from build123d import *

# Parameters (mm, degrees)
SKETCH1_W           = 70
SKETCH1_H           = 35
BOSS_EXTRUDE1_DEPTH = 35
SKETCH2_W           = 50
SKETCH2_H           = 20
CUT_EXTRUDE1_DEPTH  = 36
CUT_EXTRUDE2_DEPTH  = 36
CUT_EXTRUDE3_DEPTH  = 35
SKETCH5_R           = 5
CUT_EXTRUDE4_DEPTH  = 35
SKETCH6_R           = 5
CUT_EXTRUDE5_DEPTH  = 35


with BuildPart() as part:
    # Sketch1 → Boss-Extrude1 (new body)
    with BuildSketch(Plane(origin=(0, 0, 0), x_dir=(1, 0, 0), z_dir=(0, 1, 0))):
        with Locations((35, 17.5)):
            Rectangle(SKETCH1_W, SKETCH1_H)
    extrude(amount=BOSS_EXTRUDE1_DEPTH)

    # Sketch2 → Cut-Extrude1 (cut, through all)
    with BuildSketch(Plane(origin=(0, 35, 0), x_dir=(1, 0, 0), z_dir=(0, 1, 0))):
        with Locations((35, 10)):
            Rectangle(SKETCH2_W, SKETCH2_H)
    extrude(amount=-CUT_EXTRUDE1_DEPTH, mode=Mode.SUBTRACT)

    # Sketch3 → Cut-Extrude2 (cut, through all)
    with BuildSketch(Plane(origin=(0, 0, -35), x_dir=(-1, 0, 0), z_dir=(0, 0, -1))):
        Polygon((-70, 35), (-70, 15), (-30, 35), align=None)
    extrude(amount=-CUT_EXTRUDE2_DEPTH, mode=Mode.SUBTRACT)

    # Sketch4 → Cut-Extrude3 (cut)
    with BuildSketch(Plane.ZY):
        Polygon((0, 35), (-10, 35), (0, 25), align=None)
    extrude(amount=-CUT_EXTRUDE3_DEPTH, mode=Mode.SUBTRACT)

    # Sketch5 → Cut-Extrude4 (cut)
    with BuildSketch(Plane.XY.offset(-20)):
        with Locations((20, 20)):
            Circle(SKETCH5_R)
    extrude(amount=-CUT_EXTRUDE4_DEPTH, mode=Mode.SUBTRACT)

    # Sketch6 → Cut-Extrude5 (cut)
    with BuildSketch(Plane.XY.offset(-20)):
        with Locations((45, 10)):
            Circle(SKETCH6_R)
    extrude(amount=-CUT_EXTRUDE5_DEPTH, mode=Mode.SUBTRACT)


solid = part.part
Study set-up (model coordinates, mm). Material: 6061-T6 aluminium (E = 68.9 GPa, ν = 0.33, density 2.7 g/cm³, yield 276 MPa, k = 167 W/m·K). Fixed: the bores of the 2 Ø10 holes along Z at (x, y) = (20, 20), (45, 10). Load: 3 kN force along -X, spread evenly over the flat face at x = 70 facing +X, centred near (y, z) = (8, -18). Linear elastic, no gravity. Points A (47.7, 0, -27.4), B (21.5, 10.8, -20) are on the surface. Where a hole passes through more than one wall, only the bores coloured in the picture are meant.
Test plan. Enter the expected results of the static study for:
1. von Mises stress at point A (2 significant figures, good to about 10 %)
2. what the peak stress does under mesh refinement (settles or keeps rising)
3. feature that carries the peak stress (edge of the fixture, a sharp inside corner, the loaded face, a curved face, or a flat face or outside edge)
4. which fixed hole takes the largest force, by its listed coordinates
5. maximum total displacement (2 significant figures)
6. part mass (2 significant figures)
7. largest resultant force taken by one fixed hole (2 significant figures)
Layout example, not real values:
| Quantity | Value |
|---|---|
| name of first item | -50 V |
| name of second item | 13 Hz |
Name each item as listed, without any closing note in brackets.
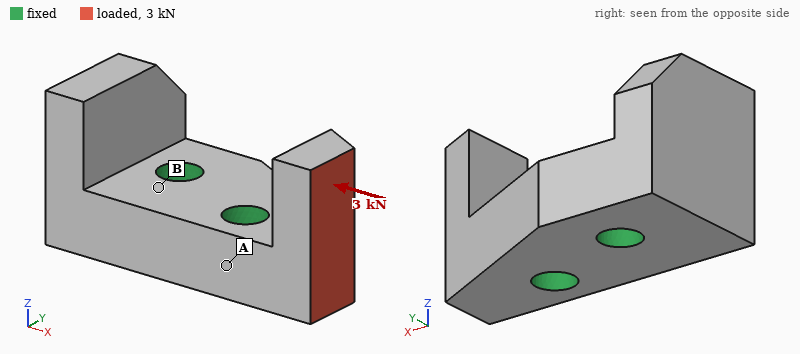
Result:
| Quantity | Value |
|---|---|
| von Mises stress at point A | 18 MPa |
| what the peak stress does under mesh refinement | keeps rising |
| feature that carries the peak stress | a sharp inside corner |
| which fixed hole takes the largest force, by its listed coordinates | (45, 10) |
| maximum total displacement | 84 µm |
| part mass | 100 g |
| largest resultant force taken by one fixed hole | 2.9 kN |
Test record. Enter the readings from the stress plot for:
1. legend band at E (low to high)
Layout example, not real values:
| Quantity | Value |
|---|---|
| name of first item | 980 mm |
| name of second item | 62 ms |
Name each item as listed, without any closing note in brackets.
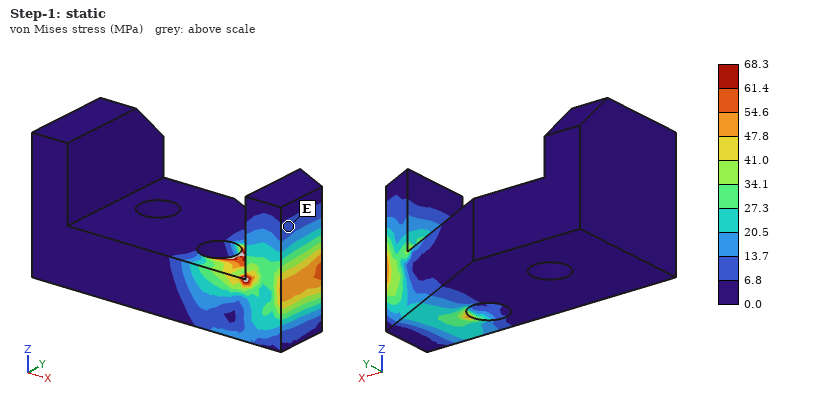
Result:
| Quantity | Value |
|---|---|
| legend band at E | 6.8 to 13.7 MPa |
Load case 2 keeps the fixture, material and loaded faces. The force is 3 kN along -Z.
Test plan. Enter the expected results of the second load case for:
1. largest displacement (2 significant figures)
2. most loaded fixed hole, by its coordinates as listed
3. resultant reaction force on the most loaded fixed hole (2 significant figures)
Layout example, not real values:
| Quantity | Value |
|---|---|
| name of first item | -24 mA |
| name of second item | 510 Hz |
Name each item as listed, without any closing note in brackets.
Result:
| Quantity | Value |
|---|---|
| largest displacement | 90 µm |
| most loaded fixed hole, by its coordinates as listed | (45, 10) |
| resultant reaction force on the most loaded fixed hole | 3.3 kN |
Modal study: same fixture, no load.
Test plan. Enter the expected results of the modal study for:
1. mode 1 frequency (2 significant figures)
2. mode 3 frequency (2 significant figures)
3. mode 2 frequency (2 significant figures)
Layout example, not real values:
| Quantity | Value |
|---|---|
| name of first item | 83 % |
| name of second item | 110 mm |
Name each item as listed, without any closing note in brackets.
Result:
| Quantity | Value |
|---|---|
| mode 1 frequency | 8800 Hz |
| mode 3 frequency | 10 kHz |
| mode 2 frequency | 9700 Hz |
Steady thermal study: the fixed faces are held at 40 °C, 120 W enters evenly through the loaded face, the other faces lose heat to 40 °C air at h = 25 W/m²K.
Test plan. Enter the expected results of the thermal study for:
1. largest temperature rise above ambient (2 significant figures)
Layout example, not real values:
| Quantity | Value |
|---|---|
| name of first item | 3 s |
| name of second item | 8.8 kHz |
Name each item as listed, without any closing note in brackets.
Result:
| Quantity | Value |
|---|---|
| largest temperature rise above ambient | 73 K |
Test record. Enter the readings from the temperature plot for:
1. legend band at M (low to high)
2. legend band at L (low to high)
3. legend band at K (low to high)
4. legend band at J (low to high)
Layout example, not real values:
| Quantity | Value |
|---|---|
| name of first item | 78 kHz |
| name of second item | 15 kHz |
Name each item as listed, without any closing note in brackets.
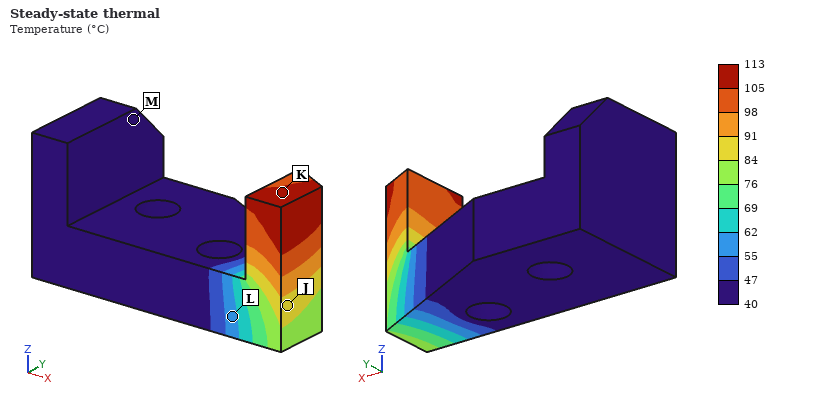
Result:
| Quantity | Value |
|---|---|
| legend band at M | 40 to 47 °C |
| legend band at L | 55 to 62 °C |
| legend band at K | 105 to 113 °C |
| legend band at J | 84 to 91 °C |
